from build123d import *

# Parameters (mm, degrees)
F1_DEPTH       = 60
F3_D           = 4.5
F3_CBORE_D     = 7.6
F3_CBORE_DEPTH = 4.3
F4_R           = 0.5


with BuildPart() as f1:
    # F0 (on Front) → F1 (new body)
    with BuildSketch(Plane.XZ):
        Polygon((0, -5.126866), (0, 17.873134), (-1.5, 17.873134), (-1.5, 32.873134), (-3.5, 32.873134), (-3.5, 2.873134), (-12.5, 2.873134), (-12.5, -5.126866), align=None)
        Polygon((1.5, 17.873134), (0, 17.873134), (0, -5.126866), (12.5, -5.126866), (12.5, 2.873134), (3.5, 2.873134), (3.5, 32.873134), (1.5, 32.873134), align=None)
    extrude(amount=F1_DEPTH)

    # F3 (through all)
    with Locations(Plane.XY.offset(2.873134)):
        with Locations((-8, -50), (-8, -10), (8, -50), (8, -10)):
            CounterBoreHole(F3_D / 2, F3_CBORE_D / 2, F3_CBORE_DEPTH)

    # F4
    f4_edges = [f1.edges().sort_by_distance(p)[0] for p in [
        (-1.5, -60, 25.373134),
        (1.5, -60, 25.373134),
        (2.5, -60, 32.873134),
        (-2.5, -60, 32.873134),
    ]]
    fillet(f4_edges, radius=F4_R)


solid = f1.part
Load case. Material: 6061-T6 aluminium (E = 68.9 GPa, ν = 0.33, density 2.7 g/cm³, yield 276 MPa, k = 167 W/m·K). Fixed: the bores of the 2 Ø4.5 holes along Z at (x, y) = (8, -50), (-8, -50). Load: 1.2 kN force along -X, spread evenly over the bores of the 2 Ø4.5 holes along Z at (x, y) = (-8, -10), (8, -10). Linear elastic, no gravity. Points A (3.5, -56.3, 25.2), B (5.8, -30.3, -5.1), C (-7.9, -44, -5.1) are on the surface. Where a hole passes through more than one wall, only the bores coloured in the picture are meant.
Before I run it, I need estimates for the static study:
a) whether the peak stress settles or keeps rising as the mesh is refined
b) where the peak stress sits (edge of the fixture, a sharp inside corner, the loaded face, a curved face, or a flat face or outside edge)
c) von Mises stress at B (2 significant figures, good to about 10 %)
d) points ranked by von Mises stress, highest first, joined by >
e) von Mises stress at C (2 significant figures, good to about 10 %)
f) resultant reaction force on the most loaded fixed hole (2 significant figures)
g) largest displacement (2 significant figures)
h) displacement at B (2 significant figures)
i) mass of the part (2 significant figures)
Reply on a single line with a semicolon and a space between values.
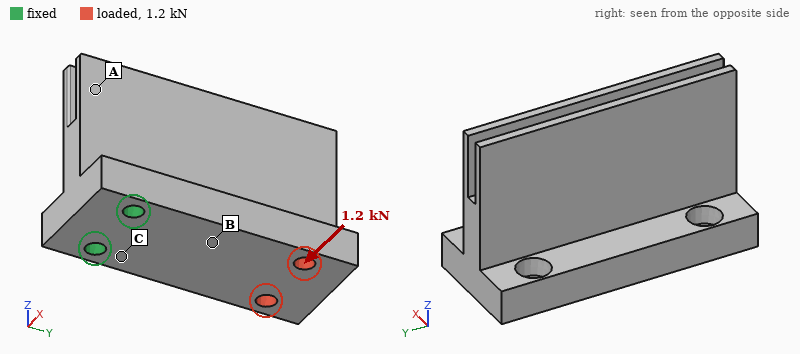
keeps rising; edge of the fixture; 26 MPa; C > B > A; 59 MPa; 2.7 kN; 84 µm; 26 µm; 56 g
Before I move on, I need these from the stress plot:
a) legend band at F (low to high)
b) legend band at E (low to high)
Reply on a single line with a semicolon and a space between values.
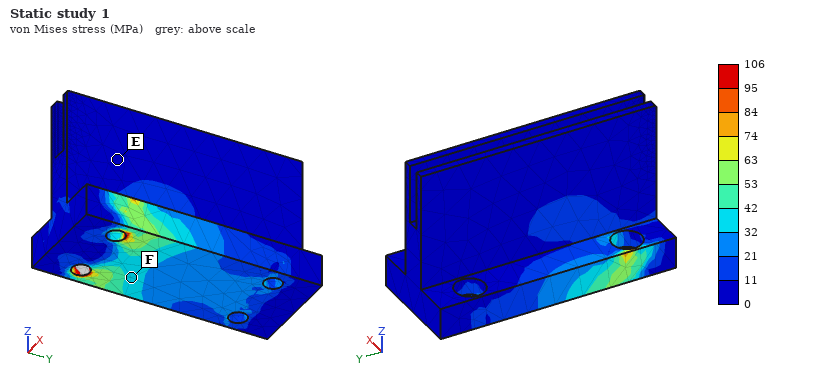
32 to 42 MPa; 0 to 11 MPa
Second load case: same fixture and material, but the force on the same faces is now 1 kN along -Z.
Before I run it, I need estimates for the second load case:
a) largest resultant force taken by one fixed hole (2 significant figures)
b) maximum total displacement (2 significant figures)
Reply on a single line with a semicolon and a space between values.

550 N; 0.39 mm
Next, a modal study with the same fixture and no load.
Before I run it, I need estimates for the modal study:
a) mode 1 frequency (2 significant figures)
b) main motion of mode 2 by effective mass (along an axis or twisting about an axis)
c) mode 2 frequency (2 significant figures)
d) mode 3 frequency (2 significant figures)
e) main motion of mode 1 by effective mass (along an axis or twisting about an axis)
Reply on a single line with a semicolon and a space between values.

1800 Hz; along X; 3500 Hz; 5200 Hz; along Z
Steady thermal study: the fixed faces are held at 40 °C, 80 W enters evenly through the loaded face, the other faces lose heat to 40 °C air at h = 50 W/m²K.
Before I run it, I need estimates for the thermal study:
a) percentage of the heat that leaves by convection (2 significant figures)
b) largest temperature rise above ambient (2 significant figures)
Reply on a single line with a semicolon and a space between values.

21 %; 78 K
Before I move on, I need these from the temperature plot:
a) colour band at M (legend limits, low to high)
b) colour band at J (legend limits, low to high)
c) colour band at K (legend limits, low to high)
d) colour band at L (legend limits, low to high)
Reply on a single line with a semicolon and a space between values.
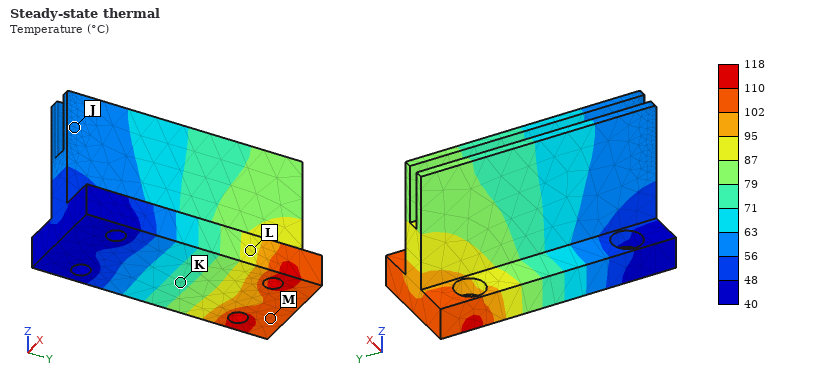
102 to 110 °C; 56 to 63 °C; 71 to 79 °C; 87 to 95 °C
